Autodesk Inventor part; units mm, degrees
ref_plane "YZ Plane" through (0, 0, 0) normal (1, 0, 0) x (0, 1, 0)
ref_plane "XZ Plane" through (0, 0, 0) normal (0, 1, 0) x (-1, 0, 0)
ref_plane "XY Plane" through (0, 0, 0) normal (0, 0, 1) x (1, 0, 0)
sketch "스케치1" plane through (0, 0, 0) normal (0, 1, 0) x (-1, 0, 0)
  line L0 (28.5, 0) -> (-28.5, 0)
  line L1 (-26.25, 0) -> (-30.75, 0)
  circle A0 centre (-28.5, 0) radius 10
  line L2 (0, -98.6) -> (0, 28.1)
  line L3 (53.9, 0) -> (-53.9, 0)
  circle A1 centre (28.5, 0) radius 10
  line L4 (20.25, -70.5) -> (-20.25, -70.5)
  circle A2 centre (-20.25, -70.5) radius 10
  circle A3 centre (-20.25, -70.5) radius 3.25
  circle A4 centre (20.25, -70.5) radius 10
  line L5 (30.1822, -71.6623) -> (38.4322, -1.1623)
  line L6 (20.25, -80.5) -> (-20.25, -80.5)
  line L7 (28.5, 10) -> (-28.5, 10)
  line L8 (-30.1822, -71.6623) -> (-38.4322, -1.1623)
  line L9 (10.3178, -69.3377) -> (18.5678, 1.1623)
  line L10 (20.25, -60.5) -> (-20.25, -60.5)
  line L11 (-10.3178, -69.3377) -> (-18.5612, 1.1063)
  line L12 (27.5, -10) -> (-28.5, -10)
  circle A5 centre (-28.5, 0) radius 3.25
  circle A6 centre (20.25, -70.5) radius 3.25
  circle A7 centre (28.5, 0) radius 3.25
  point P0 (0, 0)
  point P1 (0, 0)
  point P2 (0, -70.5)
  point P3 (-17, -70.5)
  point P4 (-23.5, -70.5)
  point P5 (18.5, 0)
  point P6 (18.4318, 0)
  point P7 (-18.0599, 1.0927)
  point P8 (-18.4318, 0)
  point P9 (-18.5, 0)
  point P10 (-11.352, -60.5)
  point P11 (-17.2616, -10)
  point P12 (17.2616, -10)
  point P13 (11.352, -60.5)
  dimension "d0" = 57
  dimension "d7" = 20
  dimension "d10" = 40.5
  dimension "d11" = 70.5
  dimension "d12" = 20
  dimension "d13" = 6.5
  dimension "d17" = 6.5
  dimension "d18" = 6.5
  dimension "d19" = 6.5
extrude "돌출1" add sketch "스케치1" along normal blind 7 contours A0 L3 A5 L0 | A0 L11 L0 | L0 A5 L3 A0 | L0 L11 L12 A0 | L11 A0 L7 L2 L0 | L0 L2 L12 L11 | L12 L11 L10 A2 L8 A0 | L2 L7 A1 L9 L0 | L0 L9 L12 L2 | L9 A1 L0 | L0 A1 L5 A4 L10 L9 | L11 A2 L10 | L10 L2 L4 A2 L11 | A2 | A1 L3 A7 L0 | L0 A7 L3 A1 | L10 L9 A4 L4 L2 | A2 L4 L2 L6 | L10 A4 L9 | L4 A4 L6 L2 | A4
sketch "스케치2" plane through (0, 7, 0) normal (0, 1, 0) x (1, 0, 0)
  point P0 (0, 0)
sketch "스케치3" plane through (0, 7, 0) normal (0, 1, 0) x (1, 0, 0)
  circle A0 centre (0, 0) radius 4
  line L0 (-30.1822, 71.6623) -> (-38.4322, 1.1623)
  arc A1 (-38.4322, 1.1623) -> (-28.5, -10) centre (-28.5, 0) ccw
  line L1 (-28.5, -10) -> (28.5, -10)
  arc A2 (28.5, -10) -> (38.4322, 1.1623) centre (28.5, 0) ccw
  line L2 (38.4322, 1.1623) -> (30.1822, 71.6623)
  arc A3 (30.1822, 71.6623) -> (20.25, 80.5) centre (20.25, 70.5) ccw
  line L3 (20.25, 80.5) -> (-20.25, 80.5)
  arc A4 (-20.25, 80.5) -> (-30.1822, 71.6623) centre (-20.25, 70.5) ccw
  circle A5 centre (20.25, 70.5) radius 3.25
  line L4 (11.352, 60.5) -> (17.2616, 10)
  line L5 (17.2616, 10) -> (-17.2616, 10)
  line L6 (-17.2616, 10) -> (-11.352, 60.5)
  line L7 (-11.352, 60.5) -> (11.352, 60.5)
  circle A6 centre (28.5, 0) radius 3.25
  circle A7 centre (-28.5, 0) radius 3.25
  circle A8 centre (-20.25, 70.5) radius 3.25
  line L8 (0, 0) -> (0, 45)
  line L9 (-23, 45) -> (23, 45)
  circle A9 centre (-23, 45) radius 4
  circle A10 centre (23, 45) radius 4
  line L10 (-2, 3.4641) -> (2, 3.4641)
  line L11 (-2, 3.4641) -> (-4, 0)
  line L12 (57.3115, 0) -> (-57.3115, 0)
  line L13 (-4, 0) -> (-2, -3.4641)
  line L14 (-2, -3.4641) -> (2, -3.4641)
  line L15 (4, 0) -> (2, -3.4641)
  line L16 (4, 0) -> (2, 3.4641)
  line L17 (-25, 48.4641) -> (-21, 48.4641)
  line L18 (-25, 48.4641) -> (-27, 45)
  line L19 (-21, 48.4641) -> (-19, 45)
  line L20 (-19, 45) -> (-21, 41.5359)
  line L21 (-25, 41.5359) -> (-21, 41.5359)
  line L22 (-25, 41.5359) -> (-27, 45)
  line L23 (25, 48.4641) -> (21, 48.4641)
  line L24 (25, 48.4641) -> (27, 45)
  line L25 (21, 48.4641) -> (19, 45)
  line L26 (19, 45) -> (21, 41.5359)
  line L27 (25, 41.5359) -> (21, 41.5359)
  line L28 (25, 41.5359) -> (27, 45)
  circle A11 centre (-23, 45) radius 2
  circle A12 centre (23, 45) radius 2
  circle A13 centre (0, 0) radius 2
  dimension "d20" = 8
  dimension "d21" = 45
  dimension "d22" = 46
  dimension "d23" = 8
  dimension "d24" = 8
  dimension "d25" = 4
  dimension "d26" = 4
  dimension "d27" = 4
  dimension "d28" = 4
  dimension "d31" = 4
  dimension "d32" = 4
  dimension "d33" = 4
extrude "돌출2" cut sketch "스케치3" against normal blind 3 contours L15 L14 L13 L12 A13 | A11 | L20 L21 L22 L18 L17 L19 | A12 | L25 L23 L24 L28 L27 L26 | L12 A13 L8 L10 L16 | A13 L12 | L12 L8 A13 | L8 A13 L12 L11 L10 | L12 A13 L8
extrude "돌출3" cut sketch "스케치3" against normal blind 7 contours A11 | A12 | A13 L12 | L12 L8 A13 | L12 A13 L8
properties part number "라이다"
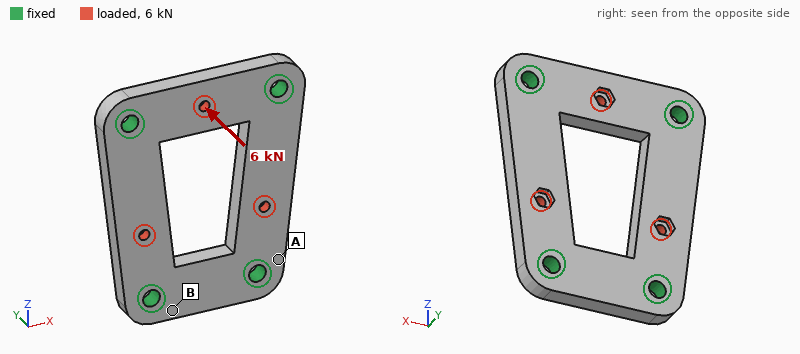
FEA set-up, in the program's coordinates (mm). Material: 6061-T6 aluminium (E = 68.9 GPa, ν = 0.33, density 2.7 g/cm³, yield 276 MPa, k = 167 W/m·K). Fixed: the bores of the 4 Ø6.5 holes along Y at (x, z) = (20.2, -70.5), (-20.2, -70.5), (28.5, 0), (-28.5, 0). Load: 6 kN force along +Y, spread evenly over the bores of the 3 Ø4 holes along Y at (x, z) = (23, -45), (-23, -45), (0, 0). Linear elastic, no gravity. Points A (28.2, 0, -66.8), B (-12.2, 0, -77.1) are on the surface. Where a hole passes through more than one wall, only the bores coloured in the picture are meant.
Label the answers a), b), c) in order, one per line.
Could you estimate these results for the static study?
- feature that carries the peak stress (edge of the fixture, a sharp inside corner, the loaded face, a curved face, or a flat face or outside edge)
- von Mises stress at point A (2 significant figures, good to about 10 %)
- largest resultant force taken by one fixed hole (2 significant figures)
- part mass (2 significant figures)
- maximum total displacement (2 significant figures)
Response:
a) the loaded face
b) 61 MPa
c) 1.6 kN
d) 85 g
e) 87 µm
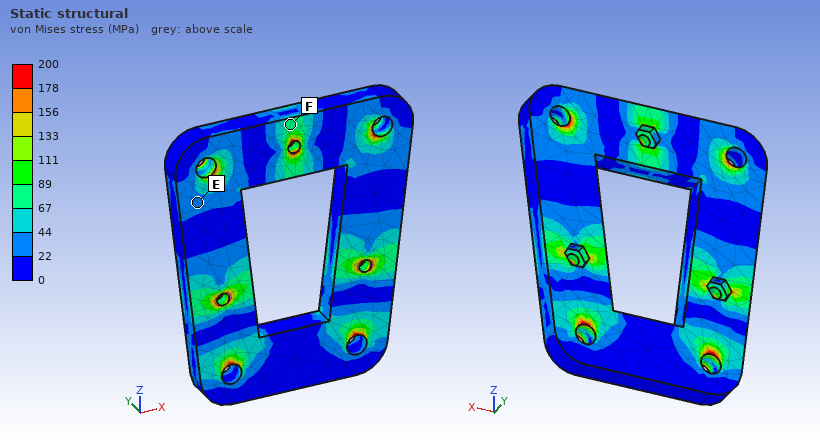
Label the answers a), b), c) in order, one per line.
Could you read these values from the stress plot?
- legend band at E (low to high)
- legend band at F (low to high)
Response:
a) 22 to 44 MPa
b) 67 to 89 MPa
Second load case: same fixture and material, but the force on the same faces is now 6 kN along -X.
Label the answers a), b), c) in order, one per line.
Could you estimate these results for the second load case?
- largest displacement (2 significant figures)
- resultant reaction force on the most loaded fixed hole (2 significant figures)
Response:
a) 23 µm
b) 1.6 kN
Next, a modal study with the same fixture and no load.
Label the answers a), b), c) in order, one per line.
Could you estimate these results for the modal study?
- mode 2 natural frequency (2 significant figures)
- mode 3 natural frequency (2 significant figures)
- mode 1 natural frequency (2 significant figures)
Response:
a) 7500 Hz
b) 11 kHz
c) 7400 Hz
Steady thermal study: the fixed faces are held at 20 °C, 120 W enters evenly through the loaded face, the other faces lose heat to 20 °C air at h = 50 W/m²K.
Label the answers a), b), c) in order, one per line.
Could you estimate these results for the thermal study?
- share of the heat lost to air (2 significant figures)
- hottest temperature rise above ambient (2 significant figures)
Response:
a) 6.1 %
b) 35 K
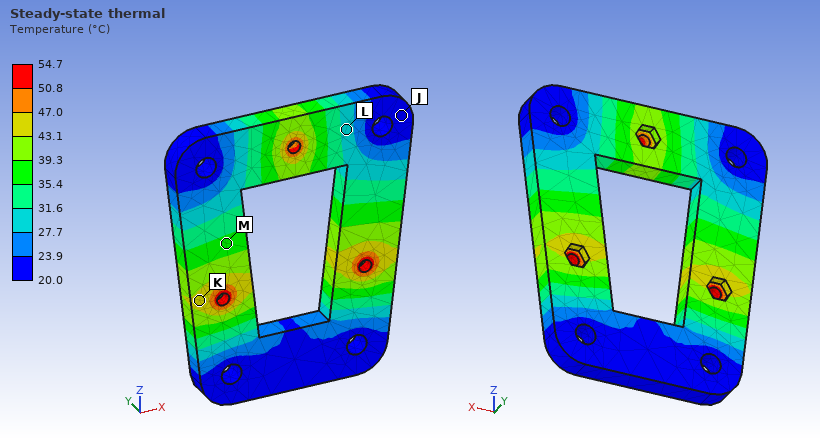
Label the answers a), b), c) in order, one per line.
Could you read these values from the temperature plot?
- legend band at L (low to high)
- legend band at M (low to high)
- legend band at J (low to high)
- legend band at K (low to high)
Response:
a) 27.7 to 31.6 °C
b) 35.4 to 39.3 °C
c) 20.0 to 23.9 °C
d) 43.1 to 47.0 °C
